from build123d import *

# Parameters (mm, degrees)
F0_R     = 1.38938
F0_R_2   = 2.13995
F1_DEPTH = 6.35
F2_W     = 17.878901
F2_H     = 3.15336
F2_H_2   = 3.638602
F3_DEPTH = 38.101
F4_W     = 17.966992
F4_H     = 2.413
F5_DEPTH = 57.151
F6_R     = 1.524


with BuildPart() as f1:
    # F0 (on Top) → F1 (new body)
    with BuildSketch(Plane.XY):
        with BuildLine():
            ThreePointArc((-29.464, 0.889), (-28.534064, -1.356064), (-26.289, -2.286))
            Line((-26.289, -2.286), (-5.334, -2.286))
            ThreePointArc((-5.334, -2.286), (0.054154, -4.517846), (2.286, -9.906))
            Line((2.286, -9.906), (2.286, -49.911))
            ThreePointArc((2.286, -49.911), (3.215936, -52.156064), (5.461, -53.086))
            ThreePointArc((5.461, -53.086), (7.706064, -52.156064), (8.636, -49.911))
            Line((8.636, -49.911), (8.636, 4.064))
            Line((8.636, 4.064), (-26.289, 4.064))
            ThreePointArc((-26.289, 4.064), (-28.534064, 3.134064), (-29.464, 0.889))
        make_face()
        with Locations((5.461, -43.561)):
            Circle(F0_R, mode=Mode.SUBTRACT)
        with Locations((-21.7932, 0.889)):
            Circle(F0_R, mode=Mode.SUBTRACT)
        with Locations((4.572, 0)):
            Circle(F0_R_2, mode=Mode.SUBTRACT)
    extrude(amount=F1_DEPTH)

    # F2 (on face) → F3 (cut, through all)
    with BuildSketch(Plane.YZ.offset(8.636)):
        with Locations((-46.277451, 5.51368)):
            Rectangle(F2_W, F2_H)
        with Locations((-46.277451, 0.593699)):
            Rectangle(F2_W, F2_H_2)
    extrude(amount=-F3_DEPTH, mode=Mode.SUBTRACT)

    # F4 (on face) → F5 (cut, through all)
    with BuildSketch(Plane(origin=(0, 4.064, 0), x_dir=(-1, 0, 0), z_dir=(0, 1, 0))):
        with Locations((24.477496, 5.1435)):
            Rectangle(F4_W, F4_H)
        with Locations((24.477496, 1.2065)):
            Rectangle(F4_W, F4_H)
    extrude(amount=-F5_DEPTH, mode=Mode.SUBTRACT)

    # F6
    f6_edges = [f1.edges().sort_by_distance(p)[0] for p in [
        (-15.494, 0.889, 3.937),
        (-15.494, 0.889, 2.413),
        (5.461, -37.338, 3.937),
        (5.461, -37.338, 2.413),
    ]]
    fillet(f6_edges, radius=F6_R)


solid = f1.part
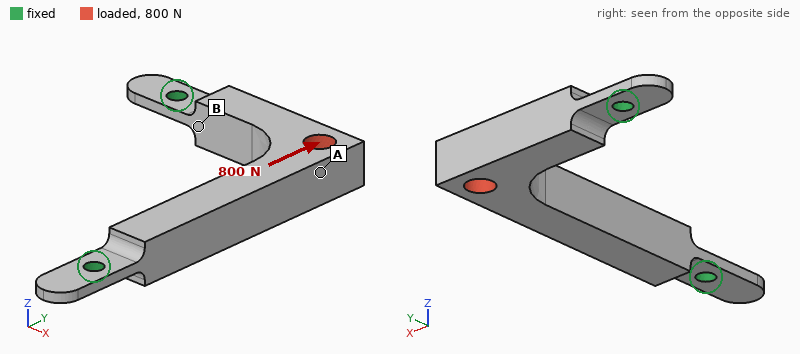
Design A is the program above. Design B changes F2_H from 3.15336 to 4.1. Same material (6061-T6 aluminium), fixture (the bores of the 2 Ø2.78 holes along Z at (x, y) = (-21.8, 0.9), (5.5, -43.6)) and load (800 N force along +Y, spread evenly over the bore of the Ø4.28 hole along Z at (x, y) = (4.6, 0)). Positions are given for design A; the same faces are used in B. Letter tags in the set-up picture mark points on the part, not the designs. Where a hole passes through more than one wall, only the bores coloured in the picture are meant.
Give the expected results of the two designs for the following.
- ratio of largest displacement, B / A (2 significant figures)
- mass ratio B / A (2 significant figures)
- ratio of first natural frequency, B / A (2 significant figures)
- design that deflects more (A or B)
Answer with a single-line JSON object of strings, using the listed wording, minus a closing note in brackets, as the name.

{"ratio of largest displacement, B / A": "2.8", "mass ratio B / A": "0.98", "ratio of first natural frequency, B / A": "0.83", "design that deflects more": "B"}
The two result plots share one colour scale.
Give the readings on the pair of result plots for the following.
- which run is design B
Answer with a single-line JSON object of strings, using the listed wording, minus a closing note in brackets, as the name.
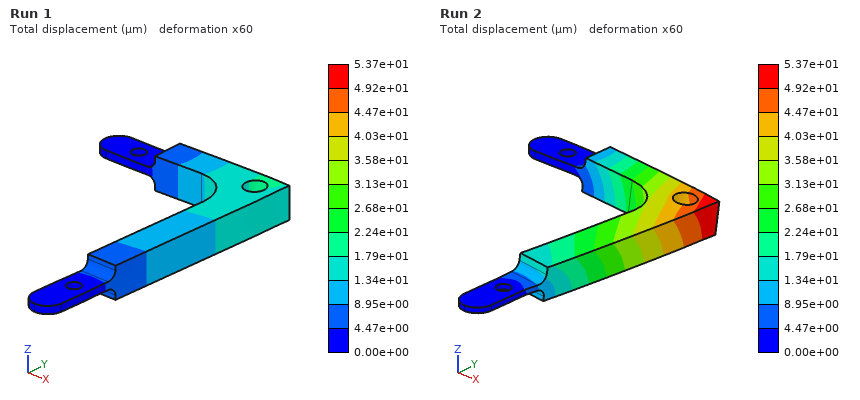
{"which run is design B": "Run 2"}
